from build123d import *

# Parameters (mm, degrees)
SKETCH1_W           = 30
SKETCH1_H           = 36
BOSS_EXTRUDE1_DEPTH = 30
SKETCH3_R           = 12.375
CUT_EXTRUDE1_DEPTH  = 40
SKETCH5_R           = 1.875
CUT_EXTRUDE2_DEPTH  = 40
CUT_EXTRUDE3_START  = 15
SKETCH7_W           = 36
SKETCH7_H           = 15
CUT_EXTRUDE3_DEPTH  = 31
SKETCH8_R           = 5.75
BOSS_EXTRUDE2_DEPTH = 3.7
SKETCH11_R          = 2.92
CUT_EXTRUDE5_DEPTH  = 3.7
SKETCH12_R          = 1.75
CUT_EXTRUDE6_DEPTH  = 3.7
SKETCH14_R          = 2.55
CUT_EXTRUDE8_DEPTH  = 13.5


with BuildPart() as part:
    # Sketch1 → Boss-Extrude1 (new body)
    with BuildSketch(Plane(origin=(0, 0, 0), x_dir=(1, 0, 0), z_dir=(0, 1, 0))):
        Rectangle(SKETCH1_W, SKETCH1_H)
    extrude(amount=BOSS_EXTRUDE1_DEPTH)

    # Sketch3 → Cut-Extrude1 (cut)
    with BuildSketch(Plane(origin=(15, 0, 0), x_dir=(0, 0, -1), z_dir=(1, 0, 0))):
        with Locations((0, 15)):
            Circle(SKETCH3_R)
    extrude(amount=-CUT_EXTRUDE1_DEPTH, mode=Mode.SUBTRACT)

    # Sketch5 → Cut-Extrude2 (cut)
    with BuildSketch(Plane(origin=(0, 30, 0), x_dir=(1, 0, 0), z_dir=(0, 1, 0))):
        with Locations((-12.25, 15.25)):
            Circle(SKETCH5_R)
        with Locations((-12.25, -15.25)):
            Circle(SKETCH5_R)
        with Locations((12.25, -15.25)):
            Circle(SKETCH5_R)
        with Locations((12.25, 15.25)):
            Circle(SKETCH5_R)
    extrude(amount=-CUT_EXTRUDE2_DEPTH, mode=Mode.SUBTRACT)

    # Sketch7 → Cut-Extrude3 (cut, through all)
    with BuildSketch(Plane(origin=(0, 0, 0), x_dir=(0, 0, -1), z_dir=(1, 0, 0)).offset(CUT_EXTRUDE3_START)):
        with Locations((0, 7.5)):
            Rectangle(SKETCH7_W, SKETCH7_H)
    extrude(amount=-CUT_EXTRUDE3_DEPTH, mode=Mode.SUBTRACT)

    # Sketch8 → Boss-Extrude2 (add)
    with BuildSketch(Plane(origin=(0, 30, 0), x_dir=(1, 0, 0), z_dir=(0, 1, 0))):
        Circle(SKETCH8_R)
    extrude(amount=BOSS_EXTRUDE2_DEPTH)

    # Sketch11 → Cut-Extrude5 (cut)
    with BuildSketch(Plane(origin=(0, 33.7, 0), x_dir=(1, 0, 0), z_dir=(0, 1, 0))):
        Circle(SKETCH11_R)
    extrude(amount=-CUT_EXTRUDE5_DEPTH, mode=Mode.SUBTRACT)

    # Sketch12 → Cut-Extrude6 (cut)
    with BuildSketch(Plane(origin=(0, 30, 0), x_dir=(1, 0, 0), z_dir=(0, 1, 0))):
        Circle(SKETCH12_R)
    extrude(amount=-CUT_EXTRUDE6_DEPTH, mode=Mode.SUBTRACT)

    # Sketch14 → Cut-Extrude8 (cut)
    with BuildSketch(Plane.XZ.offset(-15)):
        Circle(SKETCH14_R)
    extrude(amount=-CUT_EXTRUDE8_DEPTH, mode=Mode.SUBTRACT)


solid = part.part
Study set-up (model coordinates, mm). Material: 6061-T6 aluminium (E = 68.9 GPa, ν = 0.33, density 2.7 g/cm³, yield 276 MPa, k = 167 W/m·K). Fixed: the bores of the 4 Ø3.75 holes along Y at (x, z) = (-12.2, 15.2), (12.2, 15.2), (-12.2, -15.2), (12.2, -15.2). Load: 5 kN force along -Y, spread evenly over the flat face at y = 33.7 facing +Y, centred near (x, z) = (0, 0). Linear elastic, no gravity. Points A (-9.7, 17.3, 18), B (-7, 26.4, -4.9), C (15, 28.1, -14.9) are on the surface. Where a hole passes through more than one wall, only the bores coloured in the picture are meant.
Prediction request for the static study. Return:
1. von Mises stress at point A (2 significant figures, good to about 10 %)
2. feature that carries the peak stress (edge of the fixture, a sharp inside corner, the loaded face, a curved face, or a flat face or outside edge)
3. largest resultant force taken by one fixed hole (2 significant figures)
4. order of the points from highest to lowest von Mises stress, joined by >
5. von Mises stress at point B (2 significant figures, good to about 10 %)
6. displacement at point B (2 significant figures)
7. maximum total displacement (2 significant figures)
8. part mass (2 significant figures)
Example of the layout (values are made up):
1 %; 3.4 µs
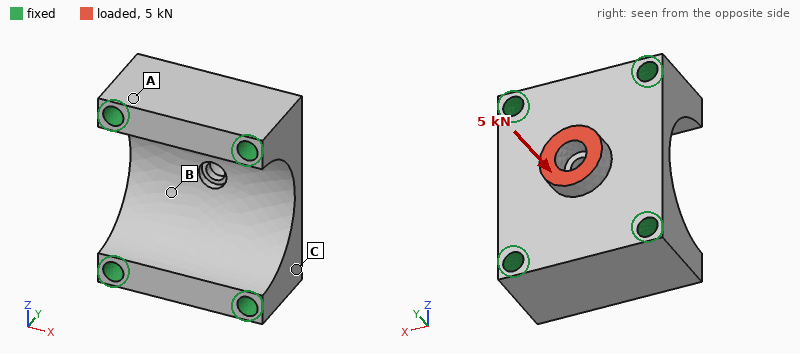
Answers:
25 MPa; a curved face; 1.8 kN; B > A > C; 70 MPa; 15 µm; 31 µm; 23 g
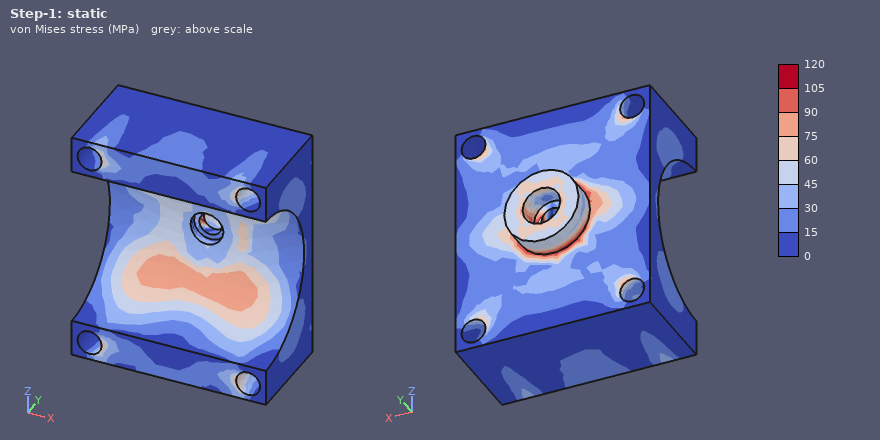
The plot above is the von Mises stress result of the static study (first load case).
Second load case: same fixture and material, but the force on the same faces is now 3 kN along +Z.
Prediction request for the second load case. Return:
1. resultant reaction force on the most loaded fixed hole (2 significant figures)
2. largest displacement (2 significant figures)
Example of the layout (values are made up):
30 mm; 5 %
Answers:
1.0 kN; 26 µm
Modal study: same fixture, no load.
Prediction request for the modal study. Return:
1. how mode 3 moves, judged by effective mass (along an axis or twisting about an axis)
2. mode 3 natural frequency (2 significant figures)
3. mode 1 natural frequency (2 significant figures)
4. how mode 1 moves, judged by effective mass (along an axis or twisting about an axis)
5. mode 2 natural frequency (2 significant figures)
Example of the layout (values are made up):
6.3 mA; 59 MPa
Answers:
along Z; 48 kHz; 37 kHz; along Y; 46 kHz
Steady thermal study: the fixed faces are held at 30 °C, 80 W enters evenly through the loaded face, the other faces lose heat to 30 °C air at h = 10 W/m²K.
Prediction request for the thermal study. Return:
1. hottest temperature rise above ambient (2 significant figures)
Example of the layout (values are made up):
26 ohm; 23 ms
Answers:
55 K
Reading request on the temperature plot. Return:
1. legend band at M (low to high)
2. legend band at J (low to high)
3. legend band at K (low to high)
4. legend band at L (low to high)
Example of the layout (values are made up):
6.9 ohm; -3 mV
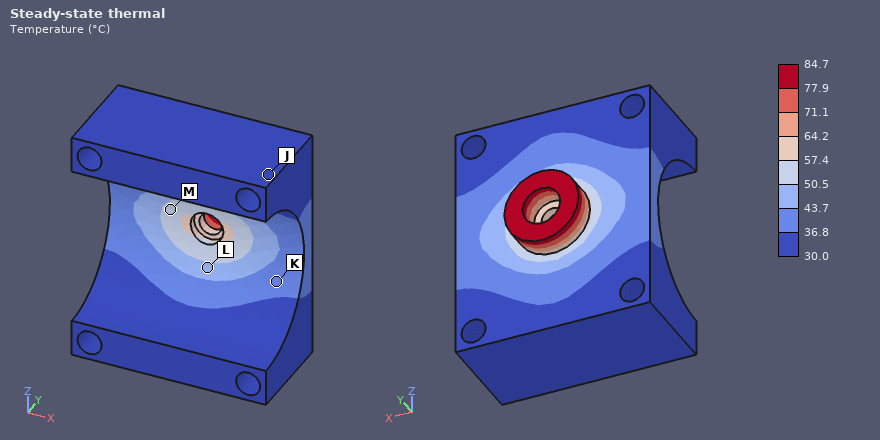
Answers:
50.5 to 57.4 °C; 30.0 to 36.8 °C; 36.8 to 43.7 °C; 43.7 to 50.5 °C
